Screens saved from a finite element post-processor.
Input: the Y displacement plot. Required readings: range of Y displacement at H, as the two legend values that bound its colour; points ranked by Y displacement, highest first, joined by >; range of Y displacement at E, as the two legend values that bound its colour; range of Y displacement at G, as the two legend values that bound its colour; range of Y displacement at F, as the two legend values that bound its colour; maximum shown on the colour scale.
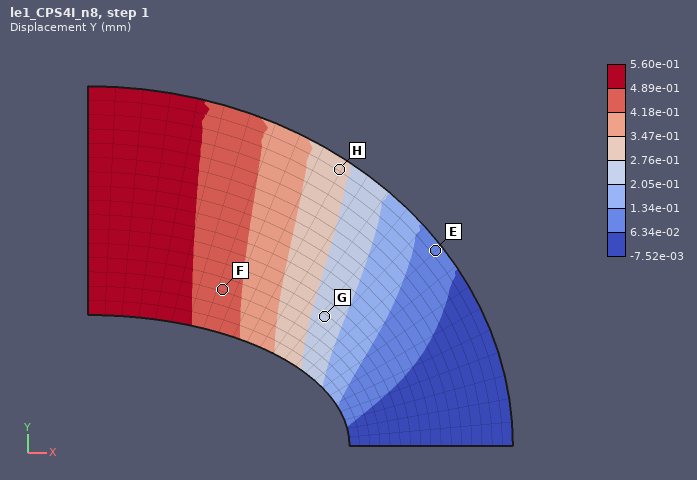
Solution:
2.76e-01 to 3.47e-01 mm
F > H > G > E
6.34e-02 to 1.34e-01 mm
2.05e-01 to 2.76e-01 mm
4.18e-01 to 4.89e-01 mm
5.60e-01 mm
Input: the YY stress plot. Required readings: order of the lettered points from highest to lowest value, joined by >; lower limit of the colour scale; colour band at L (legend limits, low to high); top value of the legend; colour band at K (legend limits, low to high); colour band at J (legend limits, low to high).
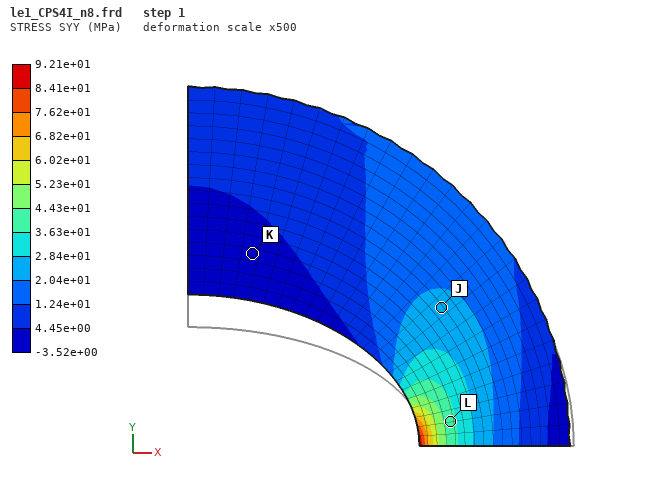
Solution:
L > J > K
-3.52e+00 MPa
3.63e+01 to 4.43e+01 MPa
9.21e+01 MPa
-3.52e+00 to 4.45e+00 MPa
2.04e+01 to 2.84e+01 MPa
